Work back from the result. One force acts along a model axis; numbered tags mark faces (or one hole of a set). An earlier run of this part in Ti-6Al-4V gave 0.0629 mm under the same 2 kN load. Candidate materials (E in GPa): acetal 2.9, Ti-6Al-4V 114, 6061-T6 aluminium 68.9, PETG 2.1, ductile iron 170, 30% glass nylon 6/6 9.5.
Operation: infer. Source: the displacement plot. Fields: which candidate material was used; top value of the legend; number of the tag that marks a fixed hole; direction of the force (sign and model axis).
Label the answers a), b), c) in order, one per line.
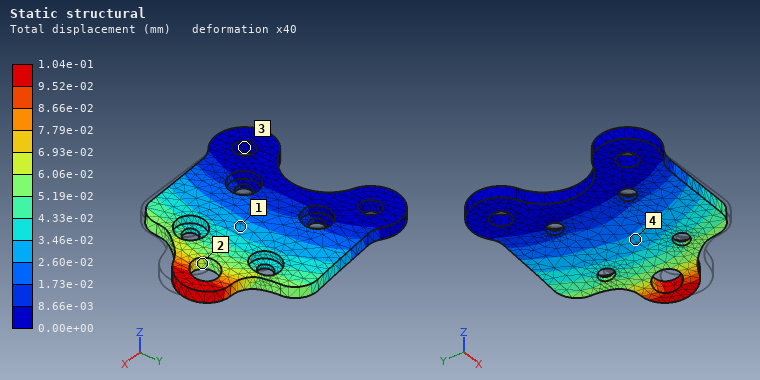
a) 6061-T6 aluminium
b) 1.04e-01 mm
c) 3
d) +Y
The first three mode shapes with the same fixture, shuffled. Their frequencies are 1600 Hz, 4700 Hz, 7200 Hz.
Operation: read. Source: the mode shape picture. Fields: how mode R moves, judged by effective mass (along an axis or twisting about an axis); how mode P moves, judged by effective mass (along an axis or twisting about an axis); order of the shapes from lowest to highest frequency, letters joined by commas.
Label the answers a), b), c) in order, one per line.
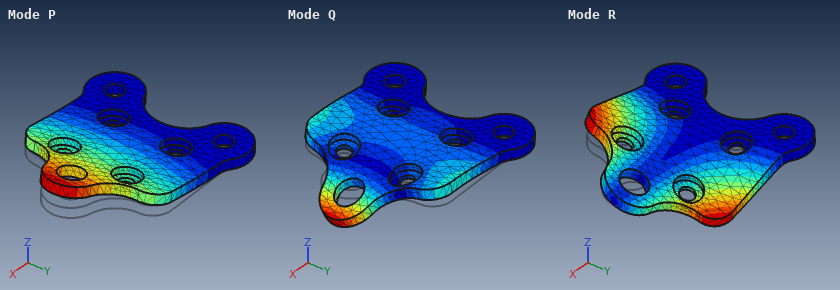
a) twisting about X
b) along Z
c) P, R, Q
